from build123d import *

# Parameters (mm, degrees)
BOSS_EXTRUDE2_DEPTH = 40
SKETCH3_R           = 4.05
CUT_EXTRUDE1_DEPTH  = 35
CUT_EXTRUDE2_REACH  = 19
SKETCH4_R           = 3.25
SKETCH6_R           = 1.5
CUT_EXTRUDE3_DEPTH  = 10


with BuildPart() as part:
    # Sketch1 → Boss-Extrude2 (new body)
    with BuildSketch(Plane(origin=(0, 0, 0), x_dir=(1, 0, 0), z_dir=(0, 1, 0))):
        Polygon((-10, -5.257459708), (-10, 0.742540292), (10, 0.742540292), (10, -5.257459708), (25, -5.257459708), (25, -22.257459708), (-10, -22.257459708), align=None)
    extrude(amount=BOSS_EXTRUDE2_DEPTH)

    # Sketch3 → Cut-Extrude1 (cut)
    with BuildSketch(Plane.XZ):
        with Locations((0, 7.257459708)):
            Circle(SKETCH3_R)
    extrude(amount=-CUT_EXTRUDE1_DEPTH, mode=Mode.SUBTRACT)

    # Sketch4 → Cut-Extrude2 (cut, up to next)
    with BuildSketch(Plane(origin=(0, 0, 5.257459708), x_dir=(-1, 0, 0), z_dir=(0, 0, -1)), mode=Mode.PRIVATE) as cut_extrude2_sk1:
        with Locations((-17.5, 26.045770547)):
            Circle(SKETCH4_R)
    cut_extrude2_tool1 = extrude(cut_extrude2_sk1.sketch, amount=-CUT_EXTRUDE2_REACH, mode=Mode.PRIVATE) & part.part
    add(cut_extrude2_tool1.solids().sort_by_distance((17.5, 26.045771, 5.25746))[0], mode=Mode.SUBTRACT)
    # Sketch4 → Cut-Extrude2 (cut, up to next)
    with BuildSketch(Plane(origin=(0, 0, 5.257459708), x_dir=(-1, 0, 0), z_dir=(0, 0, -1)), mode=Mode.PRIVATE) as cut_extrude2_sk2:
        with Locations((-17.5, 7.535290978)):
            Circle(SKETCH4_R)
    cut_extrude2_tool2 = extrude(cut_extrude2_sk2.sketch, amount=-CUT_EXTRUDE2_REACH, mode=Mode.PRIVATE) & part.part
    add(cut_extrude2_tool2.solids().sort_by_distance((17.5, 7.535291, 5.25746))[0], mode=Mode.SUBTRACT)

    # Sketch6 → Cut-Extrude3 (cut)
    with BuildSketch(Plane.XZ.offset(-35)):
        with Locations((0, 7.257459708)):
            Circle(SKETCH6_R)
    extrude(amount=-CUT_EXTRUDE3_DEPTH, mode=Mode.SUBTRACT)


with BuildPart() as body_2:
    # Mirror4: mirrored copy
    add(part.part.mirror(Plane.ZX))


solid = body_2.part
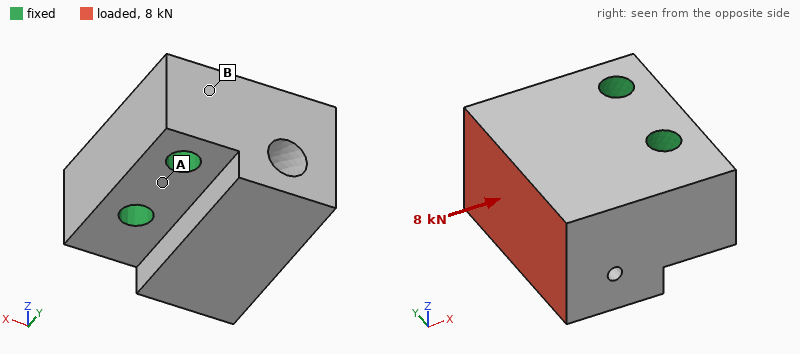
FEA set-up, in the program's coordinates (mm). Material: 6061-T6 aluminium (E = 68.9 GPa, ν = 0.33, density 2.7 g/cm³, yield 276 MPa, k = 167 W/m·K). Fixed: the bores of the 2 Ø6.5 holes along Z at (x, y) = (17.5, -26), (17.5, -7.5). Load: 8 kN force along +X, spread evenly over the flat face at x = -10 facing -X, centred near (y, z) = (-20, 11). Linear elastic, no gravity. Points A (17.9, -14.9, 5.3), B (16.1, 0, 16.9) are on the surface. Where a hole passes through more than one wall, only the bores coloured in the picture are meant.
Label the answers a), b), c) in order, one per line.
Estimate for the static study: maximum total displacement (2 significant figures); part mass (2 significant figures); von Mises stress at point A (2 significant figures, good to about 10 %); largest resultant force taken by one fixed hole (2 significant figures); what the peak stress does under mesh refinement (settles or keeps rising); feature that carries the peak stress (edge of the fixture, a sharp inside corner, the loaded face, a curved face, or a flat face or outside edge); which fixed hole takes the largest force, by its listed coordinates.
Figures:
a) 14 µm
b) 69 g
c) 8.8 MPa
d) 5.0 kN
e) keeps rising
f) edge of the fixture
g) (17.5, -26)
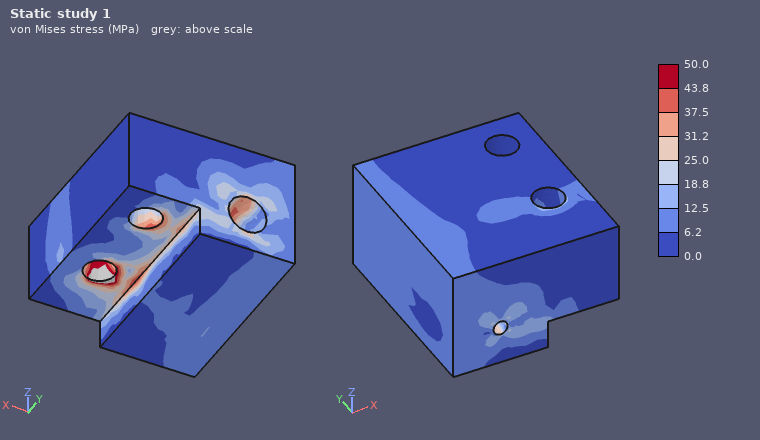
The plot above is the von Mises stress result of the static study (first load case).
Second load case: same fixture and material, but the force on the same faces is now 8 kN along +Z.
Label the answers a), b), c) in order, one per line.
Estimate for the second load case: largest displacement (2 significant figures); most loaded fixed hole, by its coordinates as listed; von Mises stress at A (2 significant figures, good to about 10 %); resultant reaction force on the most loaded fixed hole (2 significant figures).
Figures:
a) 75 µm
b) (17.5, -26)
c) 41 MPa
d) 4.7 kN
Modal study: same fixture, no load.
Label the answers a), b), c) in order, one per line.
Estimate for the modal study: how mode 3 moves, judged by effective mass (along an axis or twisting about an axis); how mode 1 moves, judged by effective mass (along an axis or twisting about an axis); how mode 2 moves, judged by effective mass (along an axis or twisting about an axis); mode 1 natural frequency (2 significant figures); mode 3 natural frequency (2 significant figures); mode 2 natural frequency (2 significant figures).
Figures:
a) twisting about X
b) along Z
c) along Y
d) 12 kHz
e) 20 kHz
f) 17 kHz
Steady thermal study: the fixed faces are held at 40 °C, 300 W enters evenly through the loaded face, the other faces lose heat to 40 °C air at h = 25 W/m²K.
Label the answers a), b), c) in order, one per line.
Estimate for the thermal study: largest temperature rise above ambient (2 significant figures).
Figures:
a) 71 K
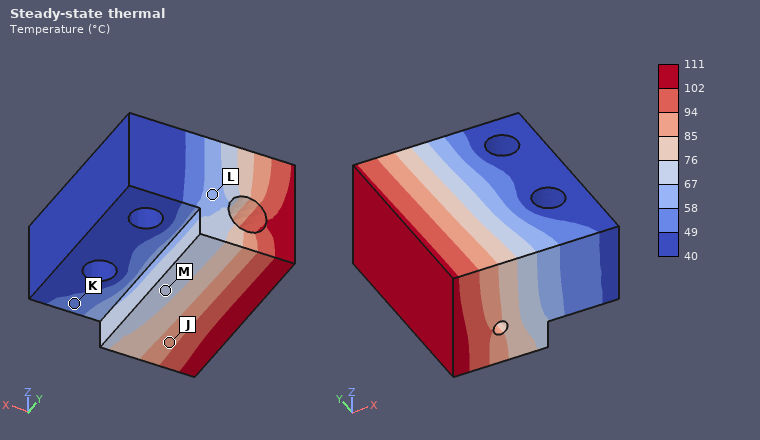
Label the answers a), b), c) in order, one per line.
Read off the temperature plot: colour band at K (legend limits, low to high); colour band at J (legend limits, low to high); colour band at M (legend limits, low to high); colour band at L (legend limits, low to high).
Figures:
a) 49 to 58 °C
b) 85 to 94 °C
c) 67 to 76 °C
d) 58 to 67 °C
